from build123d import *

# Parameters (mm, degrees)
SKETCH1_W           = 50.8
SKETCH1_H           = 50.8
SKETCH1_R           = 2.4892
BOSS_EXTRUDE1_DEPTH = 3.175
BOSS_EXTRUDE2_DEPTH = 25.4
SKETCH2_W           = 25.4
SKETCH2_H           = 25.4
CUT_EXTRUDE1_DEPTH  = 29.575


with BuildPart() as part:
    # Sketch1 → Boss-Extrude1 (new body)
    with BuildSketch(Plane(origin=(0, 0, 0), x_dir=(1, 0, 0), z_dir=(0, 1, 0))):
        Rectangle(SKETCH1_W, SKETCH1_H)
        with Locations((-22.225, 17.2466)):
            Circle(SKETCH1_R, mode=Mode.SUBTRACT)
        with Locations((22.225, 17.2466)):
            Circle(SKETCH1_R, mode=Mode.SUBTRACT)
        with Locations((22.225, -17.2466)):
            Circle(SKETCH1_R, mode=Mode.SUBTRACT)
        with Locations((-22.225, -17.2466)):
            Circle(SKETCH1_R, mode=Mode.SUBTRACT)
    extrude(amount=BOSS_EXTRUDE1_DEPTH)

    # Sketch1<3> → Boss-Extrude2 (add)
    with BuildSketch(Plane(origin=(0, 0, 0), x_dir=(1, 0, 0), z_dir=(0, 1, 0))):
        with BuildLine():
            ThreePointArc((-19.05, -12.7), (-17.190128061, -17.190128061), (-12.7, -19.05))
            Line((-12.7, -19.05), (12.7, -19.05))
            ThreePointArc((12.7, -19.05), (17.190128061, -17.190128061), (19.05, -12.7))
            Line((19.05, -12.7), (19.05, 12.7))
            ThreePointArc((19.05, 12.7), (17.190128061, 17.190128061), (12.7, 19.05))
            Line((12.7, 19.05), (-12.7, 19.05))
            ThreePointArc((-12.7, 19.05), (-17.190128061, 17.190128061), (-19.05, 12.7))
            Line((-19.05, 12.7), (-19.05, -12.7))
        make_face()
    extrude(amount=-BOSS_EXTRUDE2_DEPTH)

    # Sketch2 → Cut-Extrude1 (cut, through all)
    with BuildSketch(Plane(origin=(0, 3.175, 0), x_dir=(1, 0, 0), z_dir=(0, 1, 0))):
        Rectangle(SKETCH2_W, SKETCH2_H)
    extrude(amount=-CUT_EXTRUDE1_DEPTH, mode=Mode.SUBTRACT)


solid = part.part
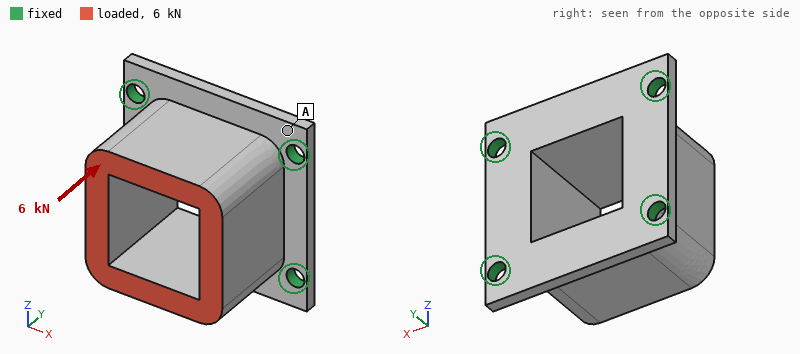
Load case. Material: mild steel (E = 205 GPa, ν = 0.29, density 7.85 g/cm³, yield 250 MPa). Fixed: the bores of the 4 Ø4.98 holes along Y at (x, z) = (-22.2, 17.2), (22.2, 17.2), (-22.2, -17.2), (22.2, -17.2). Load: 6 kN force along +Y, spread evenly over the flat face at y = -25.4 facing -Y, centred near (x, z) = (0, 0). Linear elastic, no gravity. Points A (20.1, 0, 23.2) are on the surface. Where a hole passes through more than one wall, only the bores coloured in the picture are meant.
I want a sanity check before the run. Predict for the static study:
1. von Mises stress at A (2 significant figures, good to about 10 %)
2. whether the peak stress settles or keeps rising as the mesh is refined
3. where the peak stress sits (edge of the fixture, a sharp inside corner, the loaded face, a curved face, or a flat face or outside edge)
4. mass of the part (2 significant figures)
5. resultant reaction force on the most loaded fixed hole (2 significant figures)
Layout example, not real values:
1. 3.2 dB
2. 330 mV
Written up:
1. 22 MPa
2. keeps rising
3. edge of the fixture
4. 200 g
5. 1.7 kN
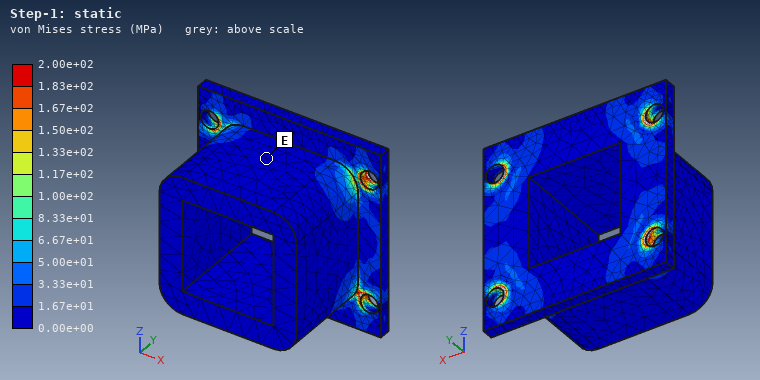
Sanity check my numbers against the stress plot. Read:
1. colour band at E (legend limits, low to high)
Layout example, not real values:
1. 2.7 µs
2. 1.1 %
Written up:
1. 0.00e+00 to 1.67e+01 MPa
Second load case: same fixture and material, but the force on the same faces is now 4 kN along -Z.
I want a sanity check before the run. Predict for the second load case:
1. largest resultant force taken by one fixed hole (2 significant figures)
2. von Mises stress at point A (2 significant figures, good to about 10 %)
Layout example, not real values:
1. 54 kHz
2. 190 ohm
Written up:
1. 2.0 kN
2. 32 MPa
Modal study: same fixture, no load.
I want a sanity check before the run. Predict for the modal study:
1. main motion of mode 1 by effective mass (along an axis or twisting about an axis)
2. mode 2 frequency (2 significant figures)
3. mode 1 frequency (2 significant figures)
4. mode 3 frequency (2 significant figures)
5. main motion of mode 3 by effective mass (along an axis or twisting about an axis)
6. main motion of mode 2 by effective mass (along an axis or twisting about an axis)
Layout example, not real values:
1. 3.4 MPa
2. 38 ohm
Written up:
1. along Z
2. 11 kHz
3. 8800 Hz
4. 12 kHz
5. along Y
6. along X
